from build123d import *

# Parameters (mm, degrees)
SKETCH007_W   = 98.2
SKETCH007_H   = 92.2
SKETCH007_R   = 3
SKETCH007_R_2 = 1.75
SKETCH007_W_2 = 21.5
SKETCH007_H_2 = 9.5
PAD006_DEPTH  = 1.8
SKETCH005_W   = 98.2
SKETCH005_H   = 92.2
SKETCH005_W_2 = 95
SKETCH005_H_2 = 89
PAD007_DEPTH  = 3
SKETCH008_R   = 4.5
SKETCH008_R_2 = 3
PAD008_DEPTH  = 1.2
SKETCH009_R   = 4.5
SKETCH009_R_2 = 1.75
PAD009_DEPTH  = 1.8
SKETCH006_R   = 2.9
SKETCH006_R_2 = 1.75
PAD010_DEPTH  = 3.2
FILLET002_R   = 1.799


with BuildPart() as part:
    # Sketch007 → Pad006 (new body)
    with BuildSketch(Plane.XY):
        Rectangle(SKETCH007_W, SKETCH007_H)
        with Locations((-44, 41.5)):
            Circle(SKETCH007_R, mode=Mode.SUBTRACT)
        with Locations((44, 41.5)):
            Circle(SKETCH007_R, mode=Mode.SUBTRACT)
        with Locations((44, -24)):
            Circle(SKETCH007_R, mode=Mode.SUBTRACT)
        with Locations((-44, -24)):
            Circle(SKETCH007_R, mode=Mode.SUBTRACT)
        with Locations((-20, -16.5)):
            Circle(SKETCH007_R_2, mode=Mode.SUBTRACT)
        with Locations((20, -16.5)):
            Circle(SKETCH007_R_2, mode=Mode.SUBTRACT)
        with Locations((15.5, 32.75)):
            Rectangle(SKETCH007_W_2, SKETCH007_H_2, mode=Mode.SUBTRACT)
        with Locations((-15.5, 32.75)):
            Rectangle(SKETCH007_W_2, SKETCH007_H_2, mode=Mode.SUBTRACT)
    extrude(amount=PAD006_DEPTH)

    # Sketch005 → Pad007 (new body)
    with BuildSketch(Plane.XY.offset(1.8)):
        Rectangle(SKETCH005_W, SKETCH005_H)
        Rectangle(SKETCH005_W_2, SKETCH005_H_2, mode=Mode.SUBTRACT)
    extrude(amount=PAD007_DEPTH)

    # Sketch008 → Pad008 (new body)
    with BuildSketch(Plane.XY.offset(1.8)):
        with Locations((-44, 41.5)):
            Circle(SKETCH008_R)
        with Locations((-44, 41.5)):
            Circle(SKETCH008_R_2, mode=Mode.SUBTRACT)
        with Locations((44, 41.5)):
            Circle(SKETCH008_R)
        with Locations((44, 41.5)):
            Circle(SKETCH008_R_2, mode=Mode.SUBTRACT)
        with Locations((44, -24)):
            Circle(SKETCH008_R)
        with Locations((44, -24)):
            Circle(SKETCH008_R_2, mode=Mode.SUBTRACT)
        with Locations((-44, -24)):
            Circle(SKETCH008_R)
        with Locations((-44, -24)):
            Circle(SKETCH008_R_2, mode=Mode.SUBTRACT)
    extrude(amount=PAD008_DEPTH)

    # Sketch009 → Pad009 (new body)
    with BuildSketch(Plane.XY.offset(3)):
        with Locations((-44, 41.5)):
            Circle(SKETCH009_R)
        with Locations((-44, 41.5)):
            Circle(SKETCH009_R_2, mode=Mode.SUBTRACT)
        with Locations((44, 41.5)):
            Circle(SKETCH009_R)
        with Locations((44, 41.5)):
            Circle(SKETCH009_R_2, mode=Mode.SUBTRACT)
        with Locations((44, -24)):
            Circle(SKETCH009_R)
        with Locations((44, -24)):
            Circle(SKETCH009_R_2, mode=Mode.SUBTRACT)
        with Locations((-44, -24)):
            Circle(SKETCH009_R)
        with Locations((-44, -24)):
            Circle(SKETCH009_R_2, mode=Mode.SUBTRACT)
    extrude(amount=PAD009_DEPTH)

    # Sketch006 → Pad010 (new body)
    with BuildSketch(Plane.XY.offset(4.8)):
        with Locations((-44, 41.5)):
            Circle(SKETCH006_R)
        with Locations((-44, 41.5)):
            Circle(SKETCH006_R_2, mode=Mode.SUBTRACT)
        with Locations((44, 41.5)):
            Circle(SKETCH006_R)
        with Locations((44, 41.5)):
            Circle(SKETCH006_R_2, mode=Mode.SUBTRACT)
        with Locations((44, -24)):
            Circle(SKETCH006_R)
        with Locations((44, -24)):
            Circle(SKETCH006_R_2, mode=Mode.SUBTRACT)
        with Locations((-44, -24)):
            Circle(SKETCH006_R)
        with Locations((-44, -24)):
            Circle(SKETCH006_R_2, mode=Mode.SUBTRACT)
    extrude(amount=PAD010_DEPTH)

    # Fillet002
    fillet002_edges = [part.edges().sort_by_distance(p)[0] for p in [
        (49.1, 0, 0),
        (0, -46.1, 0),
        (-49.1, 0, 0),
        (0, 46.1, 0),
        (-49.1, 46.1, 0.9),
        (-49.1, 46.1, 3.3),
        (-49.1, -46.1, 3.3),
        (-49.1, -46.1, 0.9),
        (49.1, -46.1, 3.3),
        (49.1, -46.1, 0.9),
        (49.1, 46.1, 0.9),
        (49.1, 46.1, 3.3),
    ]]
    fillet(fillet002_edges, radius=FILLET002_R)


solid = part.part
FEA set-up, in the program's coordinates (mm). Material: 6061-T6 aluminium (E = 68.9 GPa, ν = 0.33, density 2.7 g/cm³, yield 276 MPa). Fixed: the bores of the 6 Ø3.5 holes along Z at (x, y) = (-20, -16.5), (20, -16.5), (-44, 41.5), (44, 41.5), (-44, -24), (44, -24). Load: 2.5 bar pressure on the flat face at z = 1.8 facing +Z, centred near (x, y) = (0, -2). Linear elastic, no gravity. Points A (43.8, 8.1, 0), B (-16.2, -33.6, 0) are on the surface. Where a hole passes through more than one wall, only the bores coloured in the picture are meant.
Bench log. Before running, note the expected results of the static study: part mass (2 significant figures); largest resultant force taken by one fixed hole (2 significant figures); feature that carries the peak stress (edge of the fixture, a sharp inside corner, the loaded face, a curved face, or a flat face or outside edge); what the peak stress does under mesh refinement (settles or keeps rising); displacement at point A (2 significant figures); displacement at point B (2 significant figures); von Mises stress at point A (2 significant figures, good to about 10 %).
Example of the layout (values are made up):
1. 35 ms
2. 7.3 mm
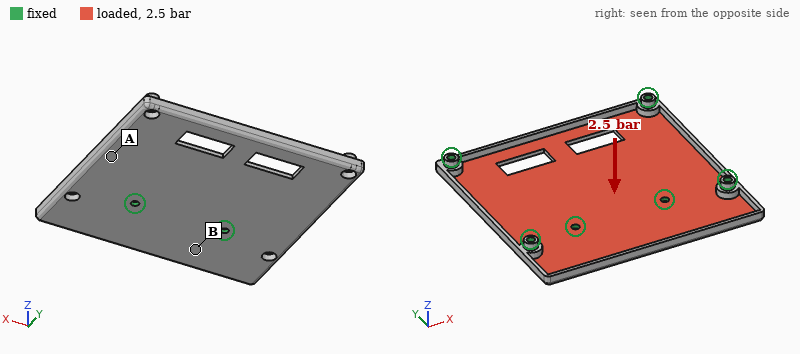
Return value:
1. 47 g
2. 540 N
3. edge of the fixture
4. keeps rising
5. 0.11 mm
6. 0.15 mm
7. 42 MPa
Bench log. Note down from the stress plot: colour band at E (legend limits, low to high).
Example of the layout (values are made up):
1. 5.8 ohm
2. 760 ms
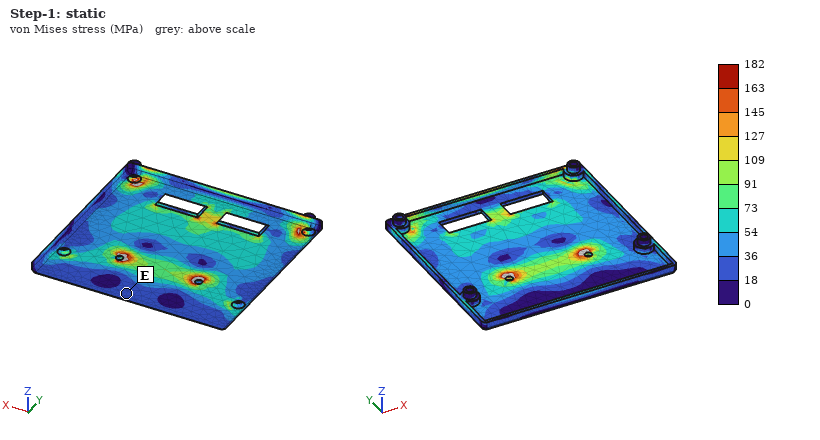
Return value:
1. 18 to 36 MPa
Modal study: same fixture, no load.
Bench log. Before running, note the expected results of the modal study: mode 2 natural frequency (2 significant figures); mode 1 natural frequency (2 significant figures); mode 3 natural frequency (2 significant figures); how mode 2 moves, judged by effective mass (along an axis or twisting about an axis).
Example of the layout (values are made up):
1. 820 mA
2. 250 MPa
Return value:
1. 2000 Hz
2. 1800 Hz
3. 3200 Hz
4. along Z
